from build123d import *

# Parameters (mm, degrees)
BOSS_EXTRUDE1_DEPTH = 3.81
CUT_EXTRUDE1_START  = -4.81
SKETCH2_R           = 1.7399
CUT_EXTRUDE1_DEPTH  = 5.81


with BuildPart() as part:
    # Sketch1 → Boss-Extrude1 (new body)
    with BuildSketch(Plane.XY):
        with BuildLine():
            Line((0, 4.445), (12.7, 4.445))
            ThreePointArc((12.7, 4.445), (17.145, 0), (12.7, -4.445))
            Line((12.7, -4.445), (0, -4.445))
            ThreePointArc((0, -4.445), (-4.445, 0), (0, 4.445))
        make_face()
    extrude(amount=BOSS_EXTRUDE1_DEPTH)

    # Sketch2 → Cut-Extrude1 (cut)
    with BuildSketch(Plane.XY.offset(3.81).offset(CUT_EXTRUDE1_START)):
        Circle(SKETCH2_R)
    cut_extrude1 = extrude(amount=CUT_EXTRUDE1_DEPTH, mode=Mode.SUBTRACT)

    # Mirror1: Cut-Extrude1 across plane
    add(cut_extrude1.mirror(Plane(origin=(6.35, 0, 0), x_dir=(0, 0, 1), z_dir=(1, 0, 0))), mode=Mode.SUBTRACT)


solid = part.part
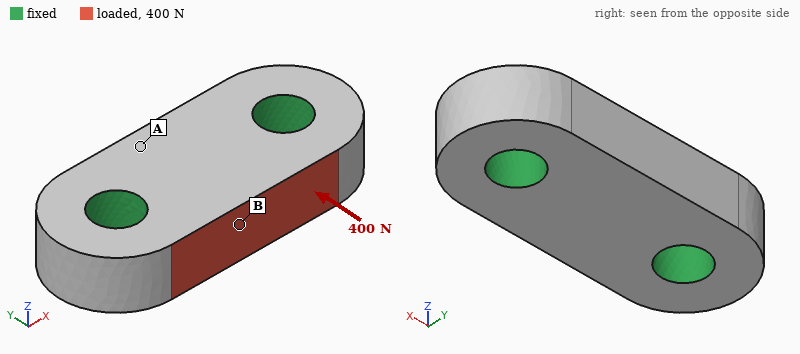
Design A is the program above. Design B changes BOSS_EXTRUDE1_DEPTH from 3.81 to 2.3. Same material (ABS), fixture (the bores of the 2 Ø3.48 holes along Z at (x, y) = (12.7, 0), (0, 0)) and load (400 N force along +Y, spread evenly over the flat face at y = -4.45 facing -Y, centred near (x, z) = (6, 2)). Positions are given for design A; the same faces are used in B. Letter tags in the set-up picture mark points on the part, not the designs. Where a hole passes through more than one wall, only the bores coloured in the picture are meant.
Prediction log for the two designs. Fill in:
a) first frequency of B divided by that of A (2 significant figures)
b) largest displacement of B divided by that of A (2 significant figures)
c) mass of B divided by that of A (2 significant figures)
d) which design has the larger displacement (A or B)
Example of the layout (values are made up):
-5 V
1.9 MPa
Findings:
0.78
1.6
0.60
B
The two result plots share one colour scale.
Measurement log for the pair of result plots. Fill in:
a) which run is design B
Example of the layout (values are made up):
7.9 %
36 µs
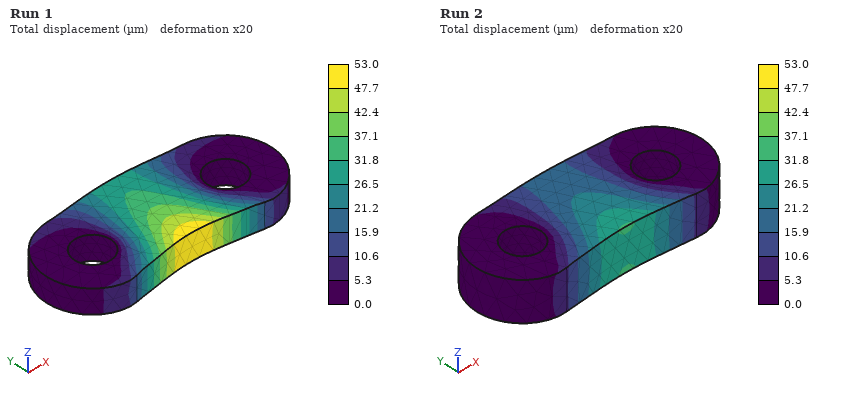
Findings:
Run 1
